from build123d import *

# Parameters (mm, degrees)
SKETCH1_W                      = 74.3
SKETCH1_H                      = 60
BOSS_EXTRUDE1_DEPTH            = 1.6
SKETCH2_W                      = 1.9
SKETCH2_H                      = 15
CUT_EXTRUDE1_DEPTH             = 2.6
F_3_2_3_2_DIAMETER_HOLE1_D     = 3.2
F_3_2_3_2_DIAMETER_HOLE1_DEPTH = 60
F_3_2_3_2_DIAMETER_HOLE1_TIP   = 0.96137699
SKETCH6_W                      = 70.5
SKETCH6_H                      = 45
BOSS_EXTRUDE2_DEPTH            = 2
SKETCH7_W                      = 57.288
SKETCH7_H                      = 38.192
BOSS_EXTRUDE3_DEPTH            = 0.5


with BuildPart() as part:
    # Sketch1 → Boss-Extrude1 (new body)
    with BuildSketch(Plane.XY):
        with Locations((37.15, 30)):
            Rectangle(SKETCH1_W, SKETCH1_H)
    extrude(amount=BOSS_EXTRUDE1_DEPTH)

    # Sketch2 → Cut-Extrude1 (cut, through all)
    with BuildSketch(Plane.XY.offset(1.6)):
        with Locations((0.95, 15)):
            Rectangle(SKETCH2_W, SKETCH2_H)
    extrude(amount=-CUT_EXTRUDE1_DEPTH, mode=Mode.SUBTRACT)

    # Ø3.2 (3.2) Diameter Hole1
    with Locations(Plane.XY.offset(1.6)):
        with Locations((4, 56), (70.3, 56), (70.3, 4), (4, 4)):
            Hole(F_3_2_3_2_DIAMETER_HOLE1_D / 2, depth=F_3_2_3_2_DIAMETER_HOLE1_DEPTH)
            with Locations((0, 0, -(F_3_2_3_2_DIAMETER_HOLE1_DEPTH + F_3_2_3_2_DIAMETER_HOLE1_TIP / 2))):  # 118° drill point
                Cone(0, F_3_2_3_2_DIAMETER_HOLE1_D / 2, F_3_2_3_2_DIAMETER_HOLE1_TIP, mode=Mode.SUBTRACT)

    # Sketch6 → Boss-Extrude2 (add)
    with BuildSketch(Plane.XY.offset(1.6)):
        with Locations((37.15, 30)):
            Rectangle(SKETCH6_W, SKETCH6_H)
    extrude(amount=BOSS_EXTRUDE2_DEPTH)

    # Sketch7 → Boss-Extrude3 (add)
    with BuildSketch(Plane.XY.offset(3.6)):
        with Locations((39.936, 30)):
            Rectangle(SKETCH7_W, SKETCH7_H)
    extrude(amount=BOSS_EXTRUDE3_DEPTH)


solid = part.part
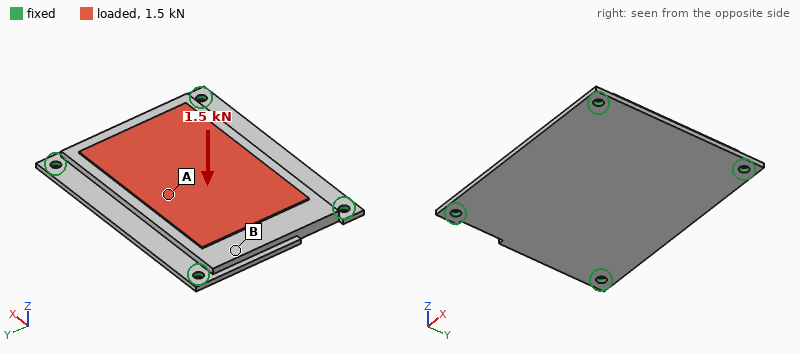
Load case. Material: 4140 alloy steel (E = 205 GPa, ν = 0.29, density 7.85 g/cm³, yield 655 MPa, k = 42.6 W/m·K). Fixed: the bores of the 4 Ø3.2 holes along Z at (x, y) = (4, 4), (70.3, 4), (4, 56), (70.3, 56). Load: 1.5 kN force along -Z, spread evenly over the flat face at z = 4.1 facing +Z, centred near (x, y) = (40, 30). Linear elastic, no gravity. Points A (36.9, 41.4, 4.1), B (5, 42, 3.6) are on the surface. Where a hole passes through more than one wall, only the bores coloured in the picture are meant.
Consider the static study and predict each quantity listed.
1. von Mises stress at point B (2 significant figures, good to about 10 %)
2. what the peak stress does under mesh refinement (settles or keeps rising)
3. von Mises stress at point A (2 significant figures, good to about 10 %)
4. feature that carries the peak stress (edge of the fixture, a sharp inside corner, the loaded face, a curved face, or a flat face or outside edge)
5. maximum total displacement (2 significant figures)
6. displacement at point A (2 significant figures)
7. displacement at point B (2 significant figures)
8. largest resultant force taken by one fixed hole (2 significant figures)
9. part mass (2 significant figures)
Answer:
35 MPa
keeps rising
71 MPa
edge of the fixture
84 µm
81 µm
21 µm
1.1 kN
110 g
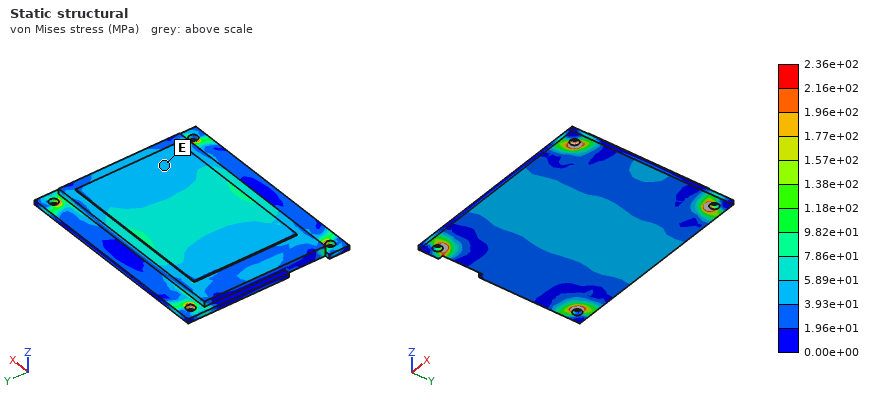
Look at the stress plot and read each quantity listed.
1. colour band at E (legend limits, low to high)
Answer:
3.93e+01 to 5.89e+01 MPa
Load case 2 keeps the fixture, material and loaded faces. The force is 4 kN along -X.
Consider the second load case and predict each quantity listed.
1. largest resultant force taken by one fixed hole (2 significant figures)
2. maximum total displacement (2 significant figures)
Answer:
1.1 kN
7.9 µm
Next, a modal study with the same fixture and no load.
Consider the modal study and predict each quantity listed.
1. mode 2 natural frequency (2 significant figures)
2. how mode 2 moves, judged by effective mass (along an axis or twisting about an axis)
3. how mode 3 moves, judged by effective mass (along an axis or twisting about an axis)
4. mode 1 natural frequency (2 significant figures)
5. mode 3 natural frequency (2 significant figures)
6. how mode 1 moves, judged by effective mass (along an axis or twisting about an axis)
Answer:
4300 Hz
twisting about X
twisting about Y
2500 Hz
5400 Hz
along Z
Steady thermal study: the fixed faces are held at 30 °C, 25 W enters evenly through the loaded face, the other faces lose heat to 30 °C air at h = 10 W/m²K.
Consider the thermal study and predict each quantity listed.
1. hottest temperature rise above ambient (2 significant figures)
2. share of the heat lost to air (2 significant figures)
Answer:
64 K
14 %
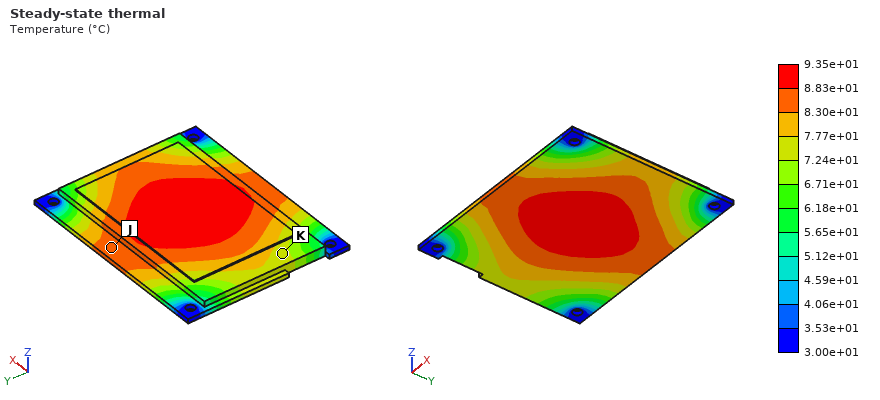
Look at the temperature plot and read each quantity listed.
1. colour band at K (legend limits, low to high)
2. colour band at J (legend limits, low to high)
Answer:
7.24e+01 to 7.77e+01 °C
8.30e+01 to 8.83e+01 °C
